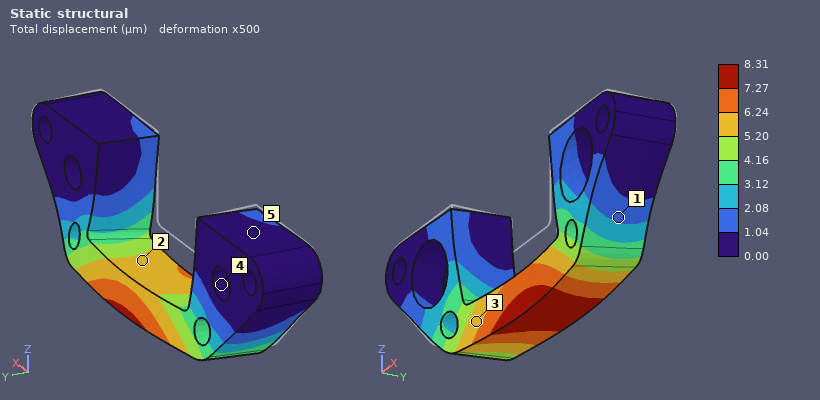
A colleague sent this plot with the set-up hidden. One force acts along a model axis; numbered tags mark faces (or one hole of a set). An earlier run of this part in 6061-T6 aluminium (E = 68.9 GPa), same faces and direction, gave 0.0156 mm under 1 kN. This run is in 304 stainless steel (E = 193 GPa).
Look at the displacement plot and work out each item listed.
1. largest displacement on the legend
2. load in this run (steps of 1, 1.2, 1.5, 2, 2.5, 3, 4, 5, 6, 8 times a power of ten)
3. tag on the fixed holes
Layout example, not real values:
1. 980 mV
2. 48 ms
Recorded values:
1. 8.31 µm
2. 1.5 kN
3. 4
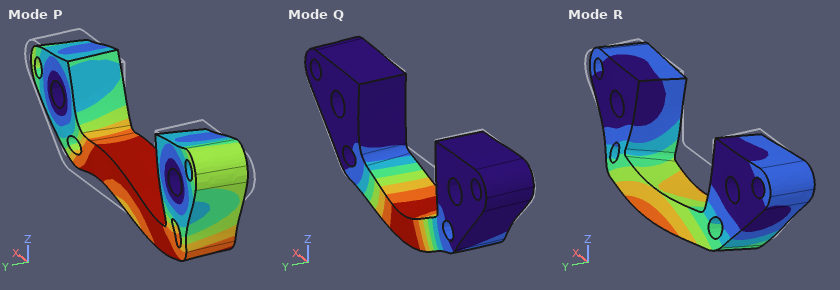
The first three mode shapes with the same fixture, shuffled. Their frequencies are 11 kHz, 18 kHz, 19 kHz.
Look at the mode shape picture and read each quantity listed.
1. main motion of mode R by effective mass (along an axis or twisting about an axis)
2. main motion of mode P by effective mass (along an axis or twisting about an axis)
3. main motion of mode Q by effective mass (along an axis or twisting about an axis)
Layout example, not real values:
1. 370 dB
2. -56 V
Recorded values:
1. along Y
2. along X
3. along Z
